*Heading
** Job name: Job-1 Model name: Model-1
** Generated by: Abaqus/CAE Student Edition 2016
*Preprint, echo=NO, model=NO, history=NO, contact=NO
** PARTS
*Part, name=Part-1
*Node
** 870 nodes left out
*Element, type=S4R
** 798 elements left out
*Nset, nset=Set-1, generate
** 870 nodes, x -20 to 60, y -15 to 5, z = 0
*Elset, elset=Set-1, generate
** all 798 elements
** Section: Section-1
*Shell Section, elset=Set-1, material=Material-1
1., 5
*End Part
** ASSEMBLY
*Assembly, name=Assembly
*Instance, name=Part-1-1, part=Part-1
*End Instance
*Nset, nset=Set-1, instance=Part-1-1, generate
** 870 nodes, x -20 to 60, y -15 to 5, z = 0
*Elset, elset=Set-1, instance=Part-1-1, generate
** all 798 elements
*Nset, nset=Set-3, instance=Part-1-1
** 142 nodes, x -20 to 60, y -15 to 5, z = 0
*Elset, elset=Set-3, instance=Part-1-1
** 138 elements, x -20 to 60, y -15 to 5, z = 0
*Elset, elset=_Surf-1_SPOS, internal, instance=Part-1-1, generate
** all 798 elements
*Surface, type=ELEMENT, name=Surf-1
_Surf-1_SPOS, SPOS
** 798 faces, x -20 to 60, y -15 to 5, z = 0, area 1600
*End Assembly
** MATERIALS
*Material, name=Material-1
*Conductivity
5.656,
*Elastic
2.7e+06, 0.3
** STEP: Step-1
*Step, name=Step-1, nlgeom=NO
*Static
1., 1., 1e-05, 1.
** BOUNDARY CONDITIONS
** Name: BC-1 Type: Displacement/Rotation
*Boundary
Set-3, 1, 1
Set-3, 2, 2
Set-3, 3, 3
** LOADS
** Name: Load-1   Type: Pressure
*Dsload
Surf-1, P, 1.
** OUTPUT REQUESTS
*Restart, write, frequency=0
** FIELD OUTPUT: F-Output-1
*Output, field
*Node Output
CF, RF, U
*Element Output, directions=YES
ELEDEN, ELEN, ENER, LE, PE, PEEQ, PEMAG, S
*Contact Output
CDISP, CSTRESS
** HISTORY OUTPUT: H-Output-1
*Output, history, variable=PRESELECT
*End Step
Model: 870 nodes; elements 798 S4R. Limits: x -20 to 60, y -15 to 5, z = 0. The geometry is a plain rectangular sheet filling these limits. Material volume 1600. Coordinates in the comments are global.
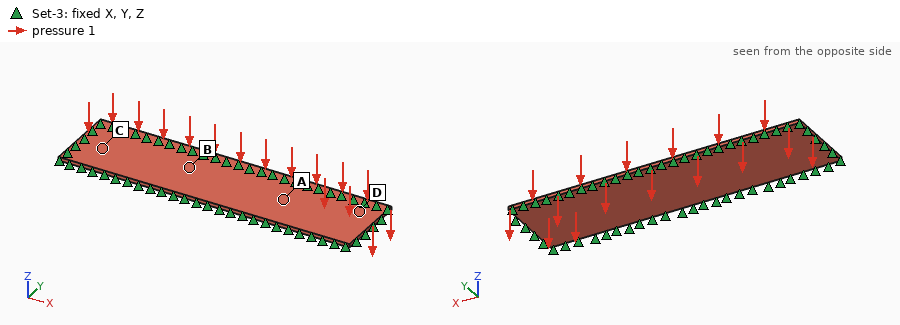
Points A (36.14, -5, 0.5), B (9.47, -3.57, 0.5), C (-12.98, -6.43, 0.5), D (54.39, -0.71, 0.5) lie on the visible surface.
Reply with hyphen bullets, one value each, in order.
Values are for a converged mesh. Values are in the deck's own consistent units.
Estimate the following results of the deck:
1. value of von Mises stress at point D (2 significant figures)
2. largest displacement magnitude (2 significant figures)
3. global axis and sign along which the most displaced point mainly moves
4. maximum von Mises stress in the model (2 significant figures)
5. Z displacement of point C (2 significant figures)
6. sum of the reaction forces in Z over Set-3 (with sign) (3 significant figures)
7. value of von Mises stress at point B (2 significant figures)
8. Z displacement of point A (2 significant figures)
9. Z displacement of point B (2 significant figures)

- 140
- 0.0084
- -Z
- 260
- -0.0041
- 1600
- 250
- -0.0079
- -0.0080
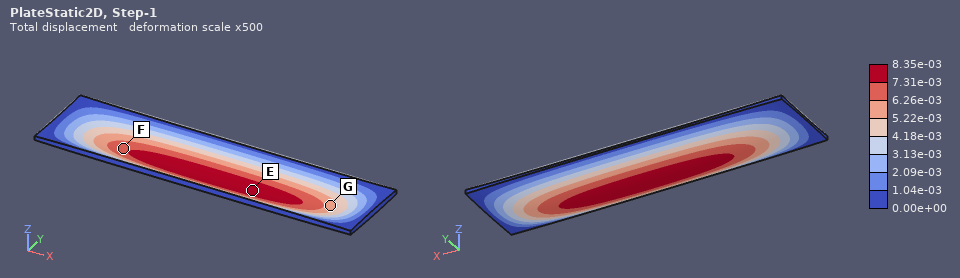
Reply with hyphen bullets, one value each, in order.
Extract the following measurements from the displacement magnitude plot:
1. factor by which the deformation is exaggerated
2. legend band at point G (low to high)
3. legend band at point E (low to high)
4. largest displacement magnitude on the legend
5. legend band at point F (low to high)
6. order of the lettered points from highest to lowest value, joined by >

- 500
- 5.22e-03 to 6.26e-03
- 7.31e-03 to 8.35e-03
- 8.35e-03
- 6.26e-03 to 7.31e-03
- E > F > G
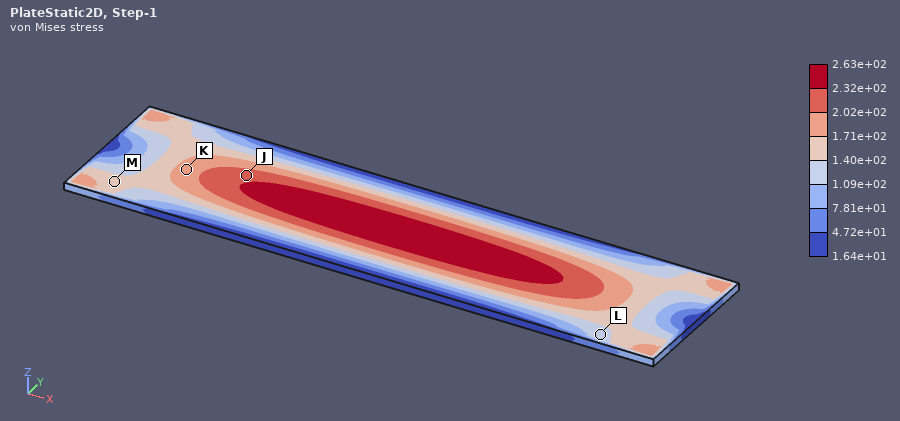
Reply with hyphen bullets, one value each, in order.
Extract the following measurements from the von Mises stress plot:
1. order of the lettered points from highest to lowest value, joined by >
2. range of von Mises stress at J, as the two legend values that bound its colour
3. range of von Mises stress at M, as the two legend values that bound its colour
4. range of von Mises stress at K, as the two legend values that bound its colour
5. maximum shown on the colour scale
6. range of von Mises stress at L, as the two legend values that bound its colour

- J > K > M > L
- 2.02e+02 to 2.32e+02
- 1.40e+02 to 1.71e+02
- 1.71e+02 to 2.02e+02
- 2.63e+02
- 1.09e+02 to 1.40e+02
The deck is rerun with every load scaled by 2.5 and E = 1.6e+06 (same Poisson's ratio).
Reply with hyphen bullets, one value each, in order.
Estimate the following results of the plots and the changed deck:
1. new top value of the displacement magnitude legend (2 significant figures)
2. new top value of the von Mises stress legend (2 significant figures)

- 0.035
- 660
